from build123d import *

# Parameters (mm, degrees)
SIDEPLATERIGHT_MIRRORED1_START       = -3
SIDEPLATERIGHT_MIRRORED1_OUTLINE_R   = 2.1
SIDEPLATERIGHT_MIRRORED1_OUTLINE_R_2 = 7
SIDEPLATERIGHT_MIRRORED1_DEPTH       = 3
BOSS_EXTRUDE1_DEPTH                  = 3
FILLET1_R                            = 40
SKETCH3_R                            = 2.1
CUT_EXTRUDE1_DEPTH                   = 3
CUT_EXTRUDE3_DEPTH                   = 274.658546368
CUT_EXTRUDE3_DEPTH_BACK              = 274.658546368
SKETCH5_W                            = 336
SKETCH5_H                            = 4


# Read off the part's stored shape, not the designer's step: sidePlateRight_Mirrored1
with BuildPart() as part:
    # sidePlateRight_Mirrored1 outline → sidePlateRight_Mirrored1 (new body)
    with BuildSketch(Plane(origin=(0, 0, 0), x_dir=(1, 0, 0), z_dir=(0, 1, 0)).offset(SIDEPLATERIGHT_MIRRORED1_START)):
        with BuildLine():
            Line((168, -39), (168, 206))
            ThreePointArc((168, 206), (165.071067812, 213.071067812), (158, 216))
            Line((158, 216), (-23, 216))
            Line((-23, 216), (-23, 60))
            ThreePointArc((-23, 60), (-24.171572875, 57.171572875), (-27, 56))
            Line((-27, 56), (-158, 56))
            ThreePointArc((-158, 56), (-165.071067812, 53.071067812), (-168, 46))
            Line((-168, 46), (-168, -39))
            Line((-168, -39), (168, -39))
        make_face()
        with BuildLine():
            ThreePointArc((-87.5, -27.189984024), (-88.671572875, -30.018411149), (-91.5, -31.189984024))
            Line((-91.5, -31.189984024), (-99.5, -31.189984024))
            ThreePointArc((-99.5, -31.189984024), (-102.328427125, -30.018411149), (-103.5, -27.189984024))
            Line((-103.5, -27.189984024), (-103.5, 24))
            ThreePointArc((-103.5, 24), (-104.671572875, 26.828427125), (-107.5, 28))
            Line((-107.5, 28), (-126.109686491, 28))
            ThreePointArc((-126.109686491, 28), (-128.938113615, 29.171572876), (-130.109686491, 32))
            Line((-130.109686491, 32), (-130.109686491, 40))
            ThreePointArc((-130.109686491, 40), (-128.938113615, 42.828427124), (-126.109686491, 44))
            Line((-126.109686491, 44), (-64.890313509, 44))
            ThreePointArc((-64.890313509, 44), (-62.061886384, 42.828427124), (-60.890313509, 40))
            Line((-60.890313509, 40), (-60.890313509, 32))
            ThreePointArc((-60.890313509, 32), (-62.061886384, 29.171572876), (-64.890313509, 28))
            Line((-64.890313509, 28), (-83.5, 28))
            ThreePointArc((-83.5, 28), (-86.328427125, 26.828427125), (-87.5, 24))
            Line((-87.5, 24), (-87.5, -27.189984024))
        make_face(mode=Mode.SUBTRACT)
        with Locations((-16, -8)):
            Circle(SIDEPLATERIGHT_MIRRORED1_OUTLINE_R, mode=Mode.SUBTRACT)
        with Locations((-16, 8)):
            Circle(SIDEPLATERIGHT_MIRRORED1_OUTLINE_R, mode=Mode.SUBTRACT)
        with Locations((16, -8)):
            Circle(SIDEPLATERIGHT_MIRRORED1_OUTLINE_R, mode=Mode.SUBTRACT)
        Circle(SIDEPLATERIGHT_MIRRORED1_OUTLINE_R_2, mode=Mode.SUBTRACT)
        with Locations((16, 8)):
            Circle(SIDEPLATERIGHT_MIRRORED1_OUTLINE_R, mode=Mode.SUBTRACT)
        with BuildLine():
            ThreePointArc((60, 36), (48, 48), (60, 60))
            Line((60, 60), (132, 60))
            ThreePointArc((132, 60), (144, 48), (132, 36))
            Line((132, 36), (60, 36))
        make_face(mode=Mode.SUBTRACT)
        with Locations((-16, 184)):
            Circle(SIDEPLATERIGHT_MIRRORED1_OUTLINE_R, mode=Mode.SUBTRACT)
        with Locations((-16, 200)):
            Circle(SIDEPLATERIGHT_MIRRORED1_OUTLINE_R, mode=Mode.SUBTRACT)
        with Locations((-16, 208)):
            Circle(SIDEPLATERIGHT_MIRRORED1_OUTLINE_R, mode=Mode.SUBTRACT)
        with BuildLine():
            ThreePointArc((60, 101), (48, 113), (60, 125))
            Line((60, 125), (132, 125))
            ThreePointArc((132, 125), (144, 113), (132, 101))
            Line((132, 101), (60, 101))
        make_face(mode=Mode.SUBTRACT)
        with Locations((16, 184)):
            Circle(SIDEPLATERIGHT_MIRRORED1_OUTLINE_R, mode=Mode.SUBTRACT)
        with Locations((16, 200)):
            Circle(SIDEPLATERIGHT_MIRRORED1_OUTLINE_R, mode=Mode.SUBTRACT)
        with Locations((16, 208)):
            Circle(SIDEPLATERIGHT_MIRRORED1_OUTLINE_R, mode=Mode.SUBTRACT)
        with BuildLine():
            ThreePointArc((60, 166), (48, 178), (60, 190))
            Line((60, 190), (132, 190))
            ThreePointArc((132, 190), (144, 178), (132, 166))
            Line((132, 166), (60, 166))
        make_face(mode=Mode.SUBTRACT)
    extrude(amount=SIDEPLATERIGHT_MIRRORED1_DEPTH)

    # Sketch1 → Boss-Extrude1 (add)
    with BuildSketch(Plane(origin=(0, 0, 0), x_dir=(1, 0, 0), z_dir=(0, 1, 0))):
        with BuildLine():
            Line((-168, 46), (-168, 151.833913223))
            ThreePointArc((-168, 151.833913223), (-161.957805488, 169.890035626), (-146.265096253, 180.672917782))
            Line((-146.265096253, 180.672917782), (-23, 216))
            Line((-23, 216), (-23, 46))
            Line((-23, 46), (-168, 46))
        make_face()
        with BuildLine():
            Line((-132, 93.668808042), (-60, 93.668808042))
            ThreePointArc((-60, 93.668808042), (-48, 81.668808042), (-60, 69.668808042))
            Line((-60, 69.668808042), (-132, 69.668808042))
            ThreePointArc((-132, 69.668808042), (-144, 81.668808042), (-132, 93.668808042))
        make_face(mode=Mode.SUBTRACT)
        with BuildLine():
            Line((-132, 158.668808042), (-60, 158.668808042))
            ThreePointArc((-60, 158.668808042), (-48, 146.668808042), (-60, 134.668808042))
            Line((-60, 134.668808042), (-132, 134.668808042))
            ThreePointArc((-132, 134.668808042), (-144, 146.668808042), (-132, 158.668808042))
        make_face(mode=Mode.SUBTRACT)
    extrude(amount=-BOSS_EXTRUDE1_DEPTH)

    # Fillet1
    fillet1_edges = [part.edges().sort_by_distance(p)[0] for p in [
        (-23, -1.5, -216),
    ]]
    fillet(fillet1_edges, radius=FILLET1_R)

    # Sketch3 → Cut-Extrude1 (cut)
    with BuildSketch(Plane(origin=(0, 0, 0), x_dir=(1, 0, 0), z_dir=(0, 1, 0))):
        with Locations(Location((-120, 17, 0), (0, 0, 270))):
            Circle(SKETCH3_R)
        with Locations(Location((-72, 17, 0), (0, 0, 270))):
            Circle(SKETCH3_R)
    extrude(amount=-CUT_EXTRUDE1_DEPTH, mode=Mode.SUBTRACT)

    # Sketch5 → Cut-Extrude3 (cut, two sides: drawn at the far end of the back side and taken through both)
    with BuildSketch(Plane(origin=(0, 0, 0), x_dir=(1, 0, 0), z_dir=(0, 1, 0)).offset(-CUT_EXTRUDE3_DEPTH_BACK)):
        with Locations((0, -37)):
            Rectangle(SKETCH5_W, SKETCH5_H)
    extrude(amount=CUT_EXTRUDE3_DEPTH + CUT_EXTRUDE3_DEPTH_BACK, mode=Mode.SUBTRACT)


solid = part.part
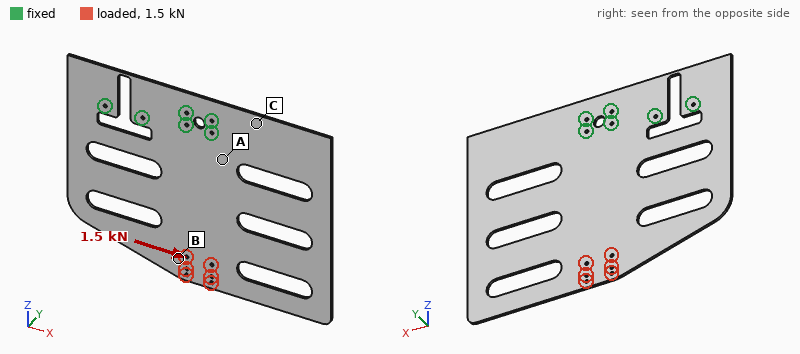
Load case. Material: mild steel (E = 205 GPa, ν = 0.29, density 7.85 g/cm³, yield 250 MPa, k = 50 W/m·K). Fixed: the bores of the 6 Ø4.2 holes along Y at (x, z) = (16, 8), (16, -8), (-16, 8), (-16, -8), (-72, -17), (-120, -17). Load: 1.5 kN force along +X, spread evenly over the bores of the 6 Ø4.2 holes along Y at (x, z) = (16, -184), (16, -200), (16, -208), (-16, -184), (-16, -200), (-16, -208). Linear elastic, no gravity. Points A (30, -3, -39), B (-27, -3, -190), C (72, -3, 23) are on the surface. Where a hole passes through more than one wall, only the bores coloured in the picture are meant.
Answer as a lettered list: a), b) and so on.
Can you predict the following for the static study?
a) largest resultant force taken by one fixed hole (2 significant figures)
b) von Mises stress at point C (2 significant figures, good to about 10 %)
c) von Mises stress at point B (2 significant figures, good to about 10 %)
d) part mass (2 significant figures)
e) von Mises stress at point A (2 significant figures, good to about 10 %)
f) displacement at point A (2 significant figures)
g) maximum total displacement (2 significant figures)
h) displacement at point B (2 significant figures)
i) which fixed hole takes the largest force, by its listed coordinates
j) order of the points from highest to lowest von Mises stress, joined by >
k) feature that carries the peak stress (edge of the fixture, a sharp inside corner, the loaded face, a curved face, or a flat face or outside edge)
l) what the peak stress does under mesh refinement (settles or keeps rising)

a) 1.9 kN
b) 3.5 MPa
c) 6.1 MPa
d) 1.6 kg
e) 12 MPa
f) 7.6 µm
g) 51 µm
h) 36 µm
i) (16, -8)
j) A > B > C
k) edge of the fixture
l) keeps rising
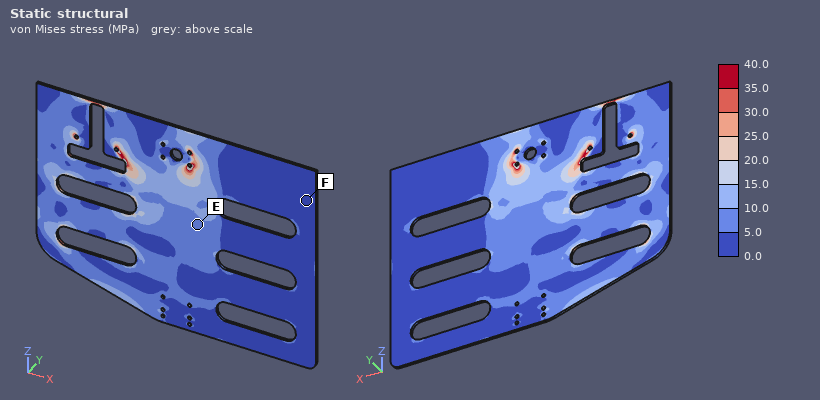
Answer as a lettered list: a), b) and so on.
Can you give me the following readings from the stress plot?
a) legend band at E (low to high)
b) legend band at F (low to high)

a) 5.0 to 10.0 MPa
b) 0.0 to 5.0 MPa
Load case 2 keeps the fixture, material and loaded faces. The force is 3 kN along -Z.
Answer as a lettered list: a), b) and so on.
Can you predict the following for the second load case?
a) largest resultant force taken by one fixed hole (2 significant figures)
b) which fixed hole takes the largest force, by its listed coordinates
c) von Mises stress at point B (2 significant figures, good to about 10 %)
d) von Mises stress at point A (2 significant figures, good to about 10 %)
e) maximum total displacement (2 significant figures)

a) 1.2 kN
b) (16, -8)
c) 10 MPa
d) 11 MPa
e) 13 µm
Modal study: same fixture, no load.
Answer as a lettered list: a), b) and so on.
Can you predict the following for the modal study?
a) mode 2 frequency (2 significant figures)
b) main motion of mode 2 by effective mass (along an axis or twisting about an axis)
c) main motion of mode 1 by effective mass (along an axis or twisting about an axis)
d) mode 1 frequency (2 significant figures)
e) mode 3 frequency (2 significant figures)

a) 79 Hz
b) twisting about Z
c) along Y
d) 46 Hz
e) 140 Hz
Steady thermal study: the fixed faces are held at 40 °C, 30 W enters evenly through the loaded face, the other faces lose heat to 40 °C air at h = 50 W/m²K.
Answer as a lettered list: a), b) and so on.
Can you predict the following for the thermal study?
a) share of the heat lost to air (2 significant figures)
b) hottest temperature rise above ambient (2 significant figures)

a) 100 %
b) 61 K
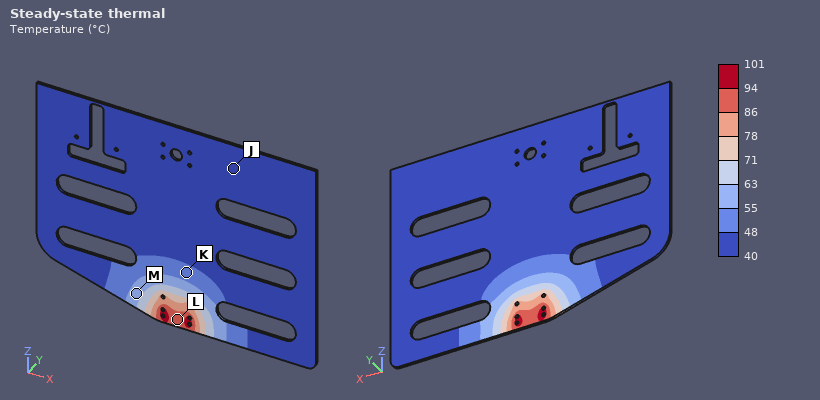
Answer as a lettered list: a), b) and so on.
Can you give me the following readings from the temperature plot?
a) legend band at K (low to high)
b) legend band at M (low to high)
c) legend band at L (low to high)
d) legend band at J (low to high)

a) 48 to 55 °C
b) 55 to 63 °C
c) 86 to 94 °C
d) 40 to 48 °C
